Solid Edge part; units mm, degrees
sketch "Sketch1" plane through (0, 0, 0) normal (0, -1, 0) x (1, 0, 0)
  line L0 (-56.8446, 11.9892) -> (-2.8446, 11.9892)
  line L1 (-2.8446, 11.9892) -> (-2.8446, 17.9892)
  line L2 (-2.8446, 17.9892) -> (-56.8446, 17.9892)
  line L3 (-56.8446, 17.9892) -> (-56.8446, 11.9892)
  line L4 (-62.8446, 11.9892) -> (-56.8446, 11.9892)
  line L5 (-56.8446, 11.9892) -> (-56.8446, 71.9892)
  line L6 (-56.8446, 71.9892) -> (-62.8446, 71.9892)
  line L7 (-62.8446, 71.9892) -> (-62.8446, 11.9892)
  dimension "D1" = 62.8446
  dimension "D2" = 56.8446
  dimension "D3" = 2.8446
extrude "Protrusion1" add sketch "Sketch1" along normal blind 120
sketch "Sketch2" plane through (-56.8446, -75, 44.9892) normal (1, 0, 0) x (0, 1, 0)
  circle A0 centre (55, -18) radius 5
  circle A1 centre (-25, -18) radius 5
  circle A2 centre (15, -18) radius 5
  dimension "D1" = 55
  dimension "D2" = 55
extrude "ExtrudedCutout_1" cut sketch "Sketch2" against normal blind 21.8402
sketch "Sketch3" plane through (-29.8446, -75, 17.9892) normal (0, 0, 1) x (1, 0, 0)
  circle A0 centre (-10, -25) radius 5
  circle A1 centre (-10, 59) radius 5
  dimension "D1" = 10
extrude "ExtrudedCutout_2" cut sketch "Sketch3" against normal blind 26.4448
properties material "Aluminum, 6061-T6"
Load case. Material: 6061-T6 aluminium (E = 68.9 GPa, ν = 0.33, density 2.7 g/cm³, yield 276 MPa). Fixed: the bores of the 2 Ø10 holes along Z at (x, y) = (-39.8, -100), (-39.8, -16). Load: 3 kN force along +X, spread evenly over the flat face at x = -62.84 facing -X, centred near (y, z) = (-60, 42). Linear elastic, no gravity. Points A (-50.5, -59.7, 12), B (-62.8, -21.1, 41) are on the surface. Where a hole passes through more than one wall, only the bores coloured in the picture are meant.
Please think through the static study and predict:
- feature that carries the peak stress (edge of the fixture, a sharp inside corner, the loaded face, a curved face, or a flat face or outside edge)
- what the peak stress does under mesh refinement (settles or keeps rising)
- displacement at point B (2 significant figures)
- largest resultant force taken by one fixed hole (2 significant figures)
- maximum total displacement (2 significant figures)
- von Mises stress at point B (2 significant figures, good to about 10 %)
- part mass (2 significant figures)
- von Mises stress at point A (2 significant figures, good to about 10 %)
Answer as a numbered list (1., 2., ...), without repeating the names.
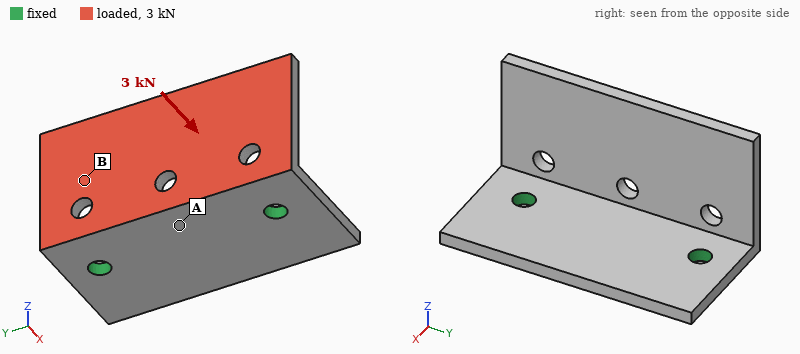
1. edge of the fixture
2. keeps rising
3. 0.44 mm
4. 1.6 kN
5. 1.1 mm
6. 27 MPa
7. 220 g
8. 73 MPa
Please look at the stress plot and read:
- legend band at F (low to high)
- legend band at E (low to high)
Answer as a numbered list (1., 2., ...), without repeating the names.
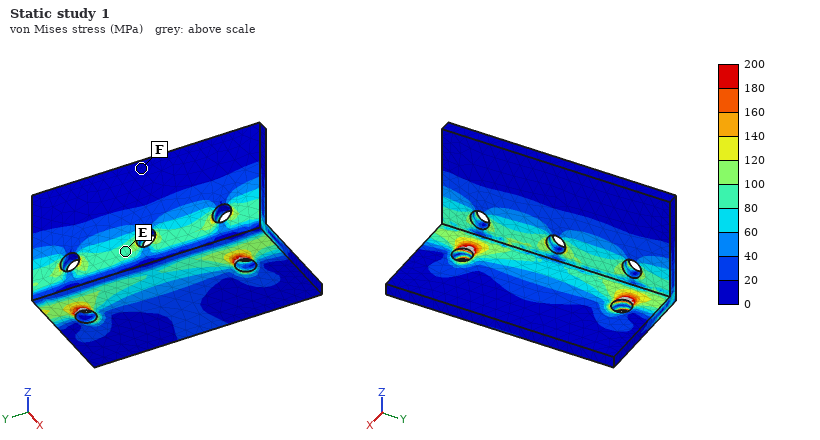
1. 0 to 20 MPa
2. 80 to 100 MPa
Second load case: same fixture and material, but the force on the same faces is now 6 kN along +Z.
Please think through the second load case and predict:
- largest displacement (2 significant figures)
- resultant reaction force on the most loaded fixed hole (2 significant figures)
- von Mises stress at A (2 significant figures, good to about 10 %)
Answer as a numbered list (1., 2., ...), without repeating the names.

1. 0.75 mm
2. 3.2 kN
3. 45 MPa
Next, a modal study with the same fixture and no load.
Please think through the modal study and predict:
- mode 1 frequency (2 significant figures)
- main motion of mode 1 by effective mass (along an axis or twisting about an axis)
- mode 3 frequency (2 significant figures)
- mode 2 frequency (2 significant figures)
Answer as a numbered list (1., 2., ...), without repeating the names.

1. 960 Hz
2. along X
3. 3000 Hz
4. 1700 Hz
